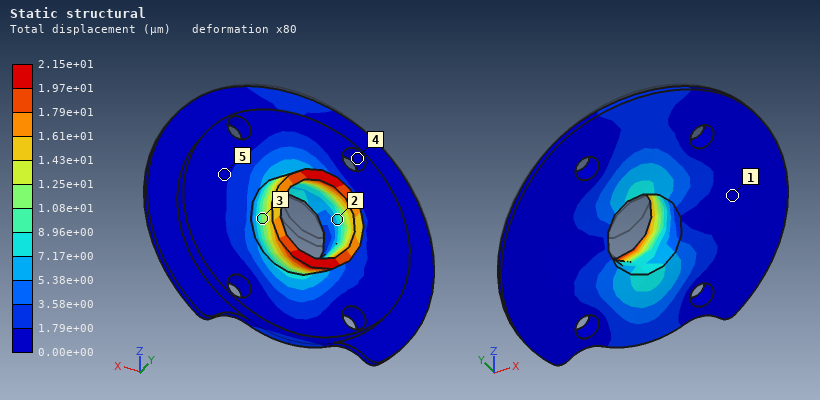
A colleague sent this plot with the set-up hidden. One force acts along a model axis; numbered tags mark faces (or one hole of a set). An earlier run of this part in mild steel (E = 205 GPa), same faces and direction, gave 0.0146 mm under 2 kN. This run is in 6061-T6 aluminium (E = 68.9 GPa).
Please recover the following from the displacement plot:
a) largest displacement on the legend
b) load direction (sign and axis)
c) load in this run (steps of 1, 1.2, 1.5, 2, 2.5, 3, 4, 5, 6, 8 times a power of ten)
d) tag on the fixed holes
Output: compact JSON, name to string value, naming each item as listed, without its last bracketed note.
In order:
{"largest displacement on the legend": "2.15e+01 µm", "load direction": "-Z", "load in this run": "1 kN", "tag on the fixed holes": "4"}
